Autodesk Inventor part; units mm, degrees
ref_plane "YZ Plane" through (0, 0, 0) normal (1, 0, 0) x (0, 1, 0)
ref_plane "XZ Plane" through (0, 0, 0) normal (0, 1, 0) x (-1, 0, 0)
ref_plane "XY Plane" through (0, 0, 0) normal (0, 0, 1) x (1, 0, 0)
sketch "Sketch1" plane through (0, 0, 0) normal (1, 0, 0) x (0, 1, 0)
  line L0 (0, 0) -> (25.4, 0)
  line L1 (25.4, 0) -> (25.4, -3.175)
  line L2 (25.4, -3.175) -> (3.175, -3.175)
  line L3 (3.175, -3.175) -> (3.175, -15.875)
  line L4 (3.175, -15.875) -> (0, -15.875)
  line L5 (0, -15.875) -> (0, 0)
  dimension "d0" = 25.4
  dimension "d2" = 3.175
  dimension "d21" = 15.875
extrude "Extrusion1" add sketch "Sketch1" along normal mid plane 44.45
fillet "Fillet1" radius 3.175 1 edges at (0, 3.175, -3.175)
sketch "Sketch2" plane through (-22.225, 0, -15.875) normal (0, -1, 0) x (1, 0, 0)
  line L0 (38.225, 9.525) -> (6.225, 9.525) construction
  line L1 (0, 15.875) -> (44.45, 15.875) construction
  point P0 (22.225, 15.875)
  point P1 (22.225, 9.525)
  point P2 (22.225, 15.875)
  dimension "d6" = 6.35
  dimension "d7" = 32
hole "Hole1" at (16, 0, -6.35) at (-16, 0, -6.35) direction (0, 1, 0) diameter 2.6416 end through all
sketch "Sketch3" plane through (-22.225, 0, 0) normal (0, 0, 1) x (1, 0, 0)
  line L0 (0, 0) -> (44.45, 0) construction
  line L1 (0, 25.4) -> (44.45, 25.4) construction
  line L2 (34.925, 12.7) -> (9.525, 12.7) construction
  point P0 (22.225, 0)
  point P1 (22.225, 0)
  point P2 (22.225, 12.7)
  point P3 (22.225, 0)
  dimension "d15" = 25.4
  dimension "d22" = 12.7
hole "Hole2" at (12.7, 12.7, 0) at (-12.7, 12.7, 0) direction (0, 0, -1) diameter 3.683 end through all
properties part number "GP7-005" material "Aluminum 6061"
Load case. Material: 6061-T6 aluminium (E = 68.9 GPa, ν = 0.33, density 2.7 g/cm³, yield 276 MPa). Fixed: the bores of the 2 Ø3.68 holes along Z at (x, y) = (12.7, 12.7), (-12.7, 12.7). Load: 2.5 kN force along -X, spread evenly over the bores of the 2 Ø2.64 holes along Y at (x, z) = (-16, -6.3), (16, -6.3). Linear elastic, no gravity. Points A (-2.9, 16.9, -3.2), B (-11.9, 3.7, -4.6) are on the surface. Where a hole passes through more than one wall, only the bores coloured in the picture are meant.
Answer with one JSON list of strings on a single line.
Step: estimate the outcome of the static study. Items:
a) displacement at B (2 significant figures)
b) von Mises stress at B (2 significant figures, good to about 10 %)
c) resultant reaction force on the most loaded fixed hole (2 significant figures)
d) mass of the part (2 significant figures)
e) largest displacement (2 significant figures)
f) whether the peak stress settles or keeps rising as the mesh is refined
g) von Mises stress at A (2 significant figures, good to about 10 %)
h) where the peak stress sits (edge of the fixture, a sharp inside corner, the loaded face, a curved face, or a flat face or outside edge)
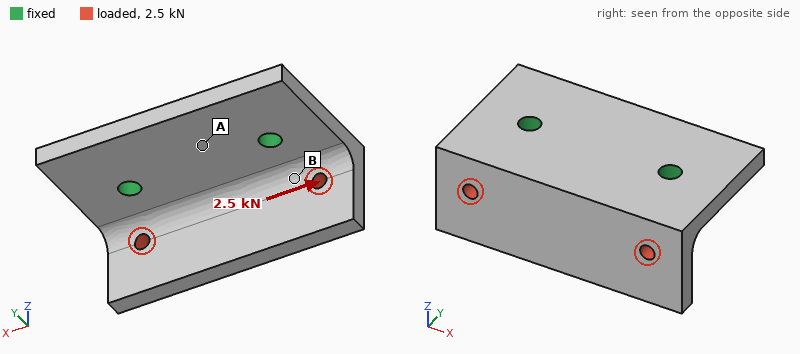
["24 µm", "82 MPa", "1.6 kN", "14 g", "66 µm", "keeps rising", "15 MPa", "edge of the fixture"]
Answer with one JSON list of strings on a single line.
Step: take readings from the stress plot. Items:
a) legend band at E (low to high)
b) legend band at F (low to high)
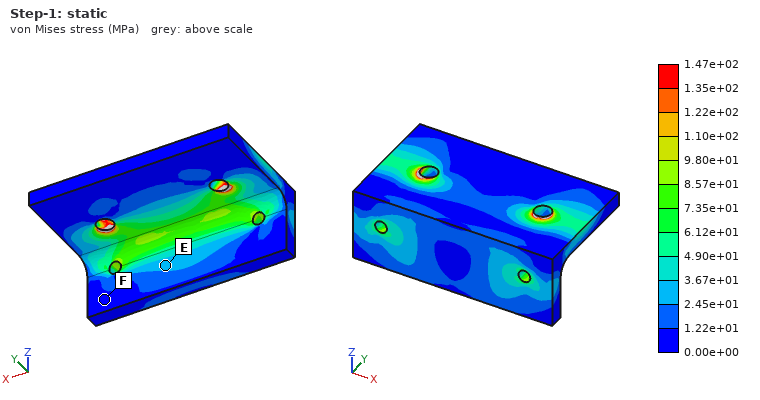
["2.45e+01 to 3.67e+01 MPa", "0.00e+00 to 1.22e+01 MPa"]
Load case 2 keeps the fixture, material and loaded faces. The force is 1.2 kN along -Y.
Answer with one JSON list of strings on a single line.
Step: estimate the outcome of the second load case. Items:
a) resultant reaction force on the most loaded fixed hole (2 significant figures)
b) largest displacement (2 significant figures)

["600 N", "0.12 mm"]
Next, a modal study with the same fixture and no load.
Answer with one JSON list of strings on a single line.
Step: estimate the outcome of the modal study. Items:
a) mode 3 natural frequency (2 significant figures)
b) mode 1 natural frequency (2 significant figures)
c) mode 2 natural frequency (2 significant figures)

["14 kHz", "5500 Hz", "8300 Hz"]
